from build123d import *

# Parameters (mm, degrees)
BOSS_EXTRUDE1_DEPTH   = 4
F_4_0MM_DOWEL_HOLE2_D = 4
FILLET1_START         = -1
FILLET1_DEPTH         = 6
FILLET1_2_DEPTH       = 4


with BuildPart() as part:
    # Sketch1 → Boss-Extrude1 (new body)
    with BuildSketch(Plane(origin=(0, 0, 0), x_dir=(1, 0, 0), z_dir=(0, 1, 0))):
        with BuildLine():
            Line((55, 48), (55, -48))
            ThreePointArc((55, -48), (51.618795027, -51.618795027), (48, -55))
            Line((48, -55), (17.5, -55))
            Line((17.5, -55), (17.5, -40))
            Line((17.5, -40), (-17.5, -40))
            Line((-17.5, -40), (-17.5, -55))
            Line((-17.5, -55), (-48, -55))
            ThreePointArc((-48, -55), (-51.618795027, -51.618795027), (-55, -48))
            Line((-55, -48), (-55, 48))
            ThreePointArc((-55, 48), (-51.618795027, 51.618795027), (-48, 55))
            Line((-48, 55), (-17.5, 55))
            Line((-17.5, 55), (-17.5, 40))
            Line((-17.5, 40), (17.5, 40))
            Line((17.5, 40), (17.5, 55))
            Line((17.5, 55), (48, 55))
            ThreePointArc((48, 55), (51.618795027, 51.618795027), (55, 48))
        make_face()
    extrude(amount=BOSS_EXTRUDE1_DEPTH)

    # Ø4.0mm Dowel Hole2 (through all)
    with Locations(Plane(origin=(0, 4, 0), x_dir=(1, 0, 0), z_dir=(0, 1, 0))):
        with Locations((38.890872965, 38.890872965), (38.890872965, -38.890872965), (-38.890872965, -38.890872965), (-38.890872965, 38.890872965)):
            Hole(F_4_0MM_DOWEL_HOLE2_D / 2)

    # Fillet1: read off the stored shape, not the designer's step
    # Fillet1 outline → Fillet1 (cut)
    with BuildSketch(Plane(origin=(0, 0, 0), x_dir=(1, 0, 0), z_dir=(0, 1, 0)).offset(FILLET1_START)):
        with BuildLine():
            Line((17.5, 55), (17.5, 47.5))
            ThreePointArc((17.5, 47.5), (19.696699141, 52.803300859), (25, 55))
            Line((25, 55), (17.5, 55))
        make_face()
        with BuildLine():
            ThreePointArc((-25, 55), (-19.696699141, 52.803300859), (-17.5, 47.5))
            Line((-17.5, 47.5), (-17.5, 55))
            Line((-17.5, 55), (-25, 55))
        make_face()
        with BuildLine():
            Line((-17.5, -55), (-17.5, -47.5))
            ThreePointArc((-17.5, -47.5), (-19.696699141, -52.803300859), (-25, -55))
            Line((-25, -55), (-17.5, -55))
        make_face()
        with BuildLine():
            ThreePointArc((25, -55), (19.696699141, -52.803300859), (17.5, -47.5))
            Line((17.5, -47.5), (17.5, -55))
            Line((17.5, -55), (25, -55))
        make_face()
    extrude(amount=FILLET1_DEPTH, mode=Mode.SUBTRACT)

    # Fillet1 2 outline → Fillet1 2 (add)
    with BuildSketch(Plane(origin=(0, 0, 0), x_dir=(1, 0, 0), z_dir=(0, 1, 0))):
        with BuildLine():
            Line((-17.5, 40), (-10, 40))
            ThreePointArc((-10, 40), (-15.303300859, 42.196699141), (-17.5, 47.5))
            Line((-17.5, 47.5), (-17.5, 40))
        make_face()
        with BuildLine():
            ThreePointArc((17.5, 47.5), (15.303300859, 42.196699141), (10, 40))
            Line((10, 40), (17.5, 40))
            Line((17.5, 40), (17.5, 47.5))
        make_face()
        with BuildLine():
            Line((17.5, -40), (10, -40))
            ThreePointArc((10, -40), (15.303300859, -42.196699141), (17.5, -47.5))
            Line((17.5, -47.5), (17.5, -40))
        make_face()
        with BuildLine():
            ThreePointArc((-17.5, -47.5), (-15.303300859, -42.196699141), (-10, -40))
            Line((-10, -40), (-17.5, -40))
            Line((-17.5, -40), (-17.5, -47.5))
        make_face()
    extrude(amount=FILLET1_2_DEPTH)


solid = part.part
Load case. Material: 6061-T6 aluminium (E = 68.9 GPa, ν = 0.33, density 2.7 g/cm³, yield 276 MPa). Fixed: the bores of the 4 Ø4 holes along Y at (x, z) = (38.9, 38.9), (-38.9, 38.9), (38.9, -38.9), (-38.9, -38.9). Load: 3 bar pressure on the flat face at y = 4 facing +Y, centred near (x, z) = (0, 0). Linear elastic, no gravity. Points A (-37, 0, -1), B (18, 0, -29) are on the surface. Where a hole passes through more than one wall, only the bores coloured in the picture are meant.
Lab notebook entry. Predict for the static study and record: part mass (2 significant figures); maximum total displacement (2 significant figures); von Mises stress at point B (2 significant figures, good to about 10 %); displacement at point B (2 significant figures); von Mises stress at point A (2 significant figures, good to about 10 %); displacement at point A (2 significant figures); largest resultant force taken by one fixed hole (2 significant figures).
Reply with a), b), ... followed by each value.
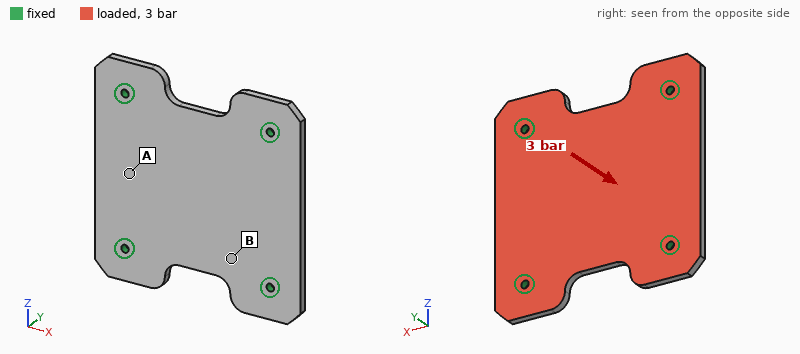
a) 120 g
b) 0.20 mm
c) 17 MPa
d) 0.099 mm
e) 35 MPa
f) 0.12 mm
g) 820 N
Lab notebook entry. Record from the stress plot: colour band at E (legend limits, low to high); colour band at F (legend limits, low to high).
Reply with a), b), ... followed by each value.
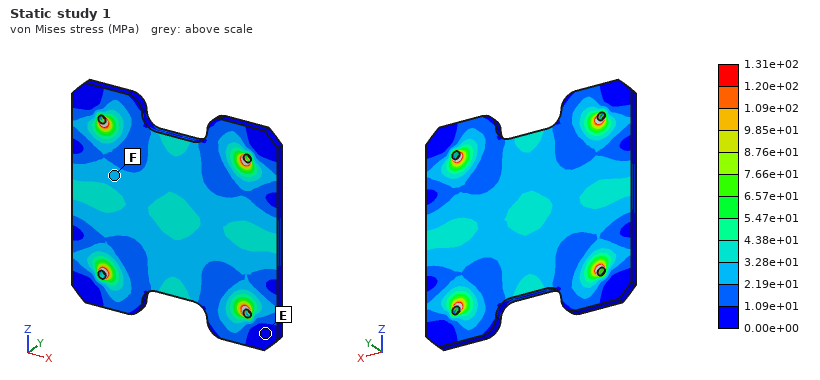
a) 0.00e+00 to 1.09e+01 MPa
b) 2.19e+01 to 3.28e+01 MPa
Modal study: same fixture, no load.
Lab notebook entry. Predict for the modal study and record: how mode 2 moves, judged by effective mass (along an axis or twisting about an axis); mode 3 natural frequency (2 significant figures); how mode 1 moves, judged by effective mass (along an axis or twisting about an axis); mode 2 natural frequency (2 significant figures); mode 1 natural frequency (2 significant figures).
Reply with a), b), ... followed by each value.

a) twisting about Z
b) 3600 Hz
c) along Y
d) 3400 Hz
e) 2300 Hz
